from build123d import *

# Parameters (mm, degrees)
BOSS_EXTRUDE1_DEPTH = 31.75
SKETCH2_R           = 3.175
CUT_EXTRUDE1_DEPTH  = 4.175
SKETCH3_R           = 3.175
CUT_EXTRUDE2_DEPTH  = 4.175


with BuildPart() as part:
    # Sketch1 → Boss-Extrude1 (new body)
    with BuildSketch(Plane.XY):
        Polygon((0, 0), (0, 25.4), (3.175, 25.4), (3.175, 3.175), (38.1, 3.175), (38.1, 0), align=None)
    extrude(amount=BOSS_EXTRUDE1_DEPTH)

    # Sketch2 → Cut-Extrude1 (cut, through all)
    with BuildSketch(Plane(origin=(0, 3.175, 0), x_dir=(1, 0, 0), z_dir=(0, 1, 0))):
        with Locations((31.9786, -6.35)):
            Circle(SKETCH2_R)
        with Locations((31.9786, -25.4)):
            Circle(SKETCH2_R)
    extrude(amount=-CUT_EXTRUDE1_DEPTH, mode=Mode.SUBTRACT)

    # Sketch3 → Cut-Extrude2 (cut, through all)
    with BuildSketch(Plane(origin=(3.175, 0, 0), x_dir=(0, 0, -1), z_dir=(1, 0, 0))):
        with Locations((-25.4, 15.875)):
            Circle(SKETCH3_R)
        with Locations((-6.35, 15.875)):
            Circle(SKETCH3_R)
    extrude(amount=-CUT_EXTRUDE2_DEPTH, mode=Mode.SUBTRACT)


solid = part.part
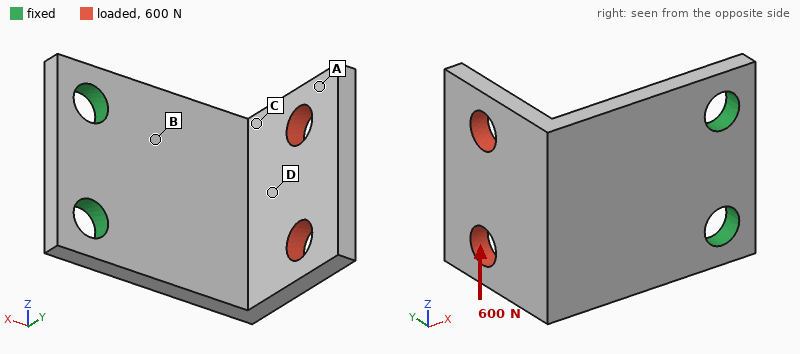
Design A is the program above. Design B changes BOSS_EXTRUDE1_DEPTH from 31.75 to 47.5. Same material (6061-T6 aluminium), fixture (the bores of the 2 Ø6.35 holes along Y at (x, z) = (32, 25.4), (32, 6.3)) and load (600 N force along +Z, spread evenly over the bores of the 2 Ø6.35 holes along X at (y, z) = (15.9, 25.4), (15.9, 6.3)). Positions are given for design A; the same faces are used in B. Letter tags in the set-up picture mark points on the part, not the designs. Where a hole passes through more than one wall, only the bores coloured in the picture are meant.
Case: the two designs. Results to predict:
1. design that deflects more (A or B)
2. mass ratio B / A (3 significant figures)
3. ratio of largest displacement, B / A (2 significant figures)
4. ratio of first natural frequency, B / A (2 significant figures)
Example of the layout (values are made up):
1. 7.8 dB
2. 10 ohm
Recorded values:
1. A
2. 1.53
3. 0.87
4. 0.92
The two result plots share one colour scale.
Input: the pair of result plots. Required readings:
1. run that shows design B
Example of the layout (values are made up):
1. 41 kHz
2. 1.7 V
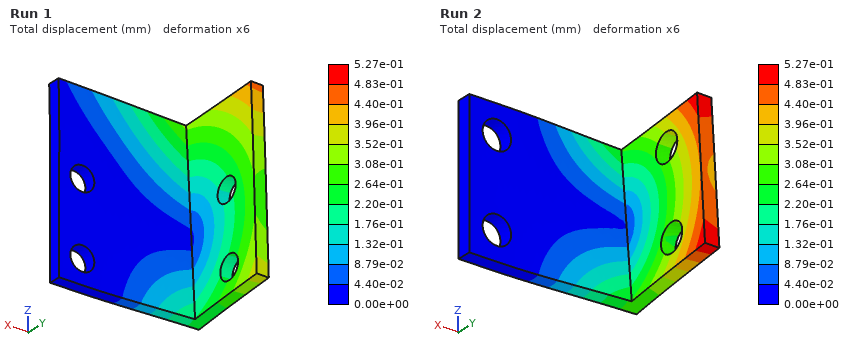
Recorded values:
1. Run 1
